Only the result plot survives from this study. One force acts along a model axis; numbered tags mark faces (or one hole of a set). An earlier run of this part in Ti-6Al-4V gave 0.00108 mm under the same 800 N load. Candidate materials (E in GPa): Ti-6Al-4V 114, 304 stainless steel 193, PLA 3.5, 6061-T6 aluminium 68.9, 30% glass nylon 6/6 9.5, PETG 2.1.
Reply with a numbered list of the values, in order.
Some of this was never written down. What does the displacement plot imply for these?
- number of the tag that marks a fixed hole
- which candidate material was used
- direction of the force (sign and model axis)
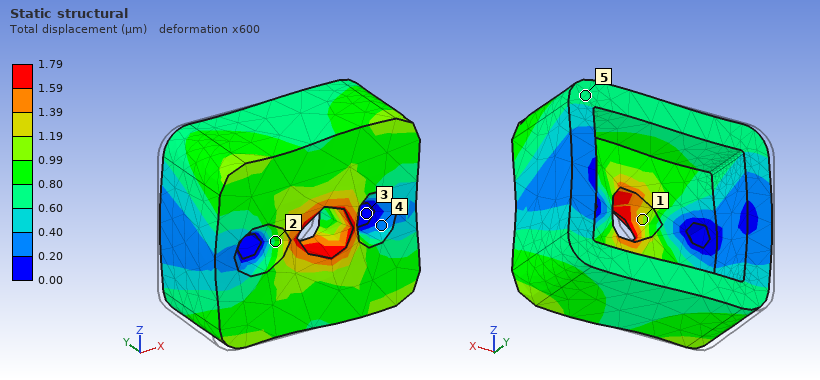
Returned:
1. 3
2. 6061-T6 aluminium
3. +X
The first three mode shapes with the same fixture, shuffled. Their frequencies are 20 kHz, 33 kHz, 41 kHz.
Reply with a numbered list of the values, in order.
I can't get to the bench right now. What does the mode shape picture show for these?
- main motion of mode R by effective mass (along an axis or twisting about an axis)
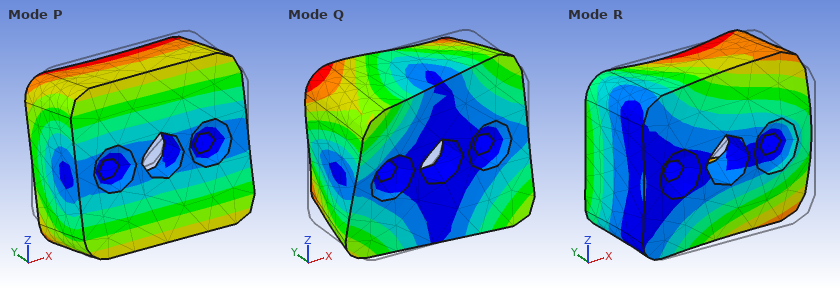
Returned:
1. along Y
